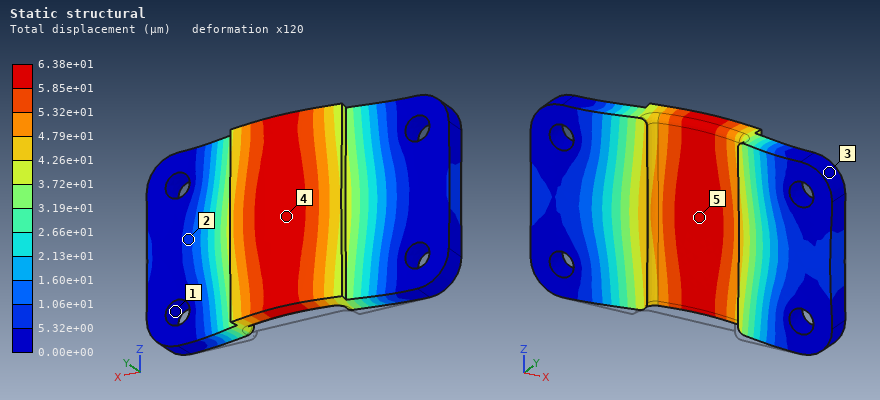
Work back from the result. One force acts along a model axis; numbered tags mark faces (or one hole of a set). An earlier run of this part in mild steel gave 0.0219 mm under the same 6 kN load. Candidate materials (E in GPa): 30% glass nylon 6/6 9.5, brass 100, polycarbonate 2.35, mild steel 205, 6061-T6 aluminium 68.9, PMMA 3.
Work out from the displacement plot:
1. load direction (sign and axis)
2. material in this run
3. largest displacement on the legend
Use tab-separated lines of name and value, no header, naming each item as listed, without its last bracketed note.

load direction	+Y
material in this run	6061-T6 aluminium
largest displacement on the legend	6.38e+01 µm
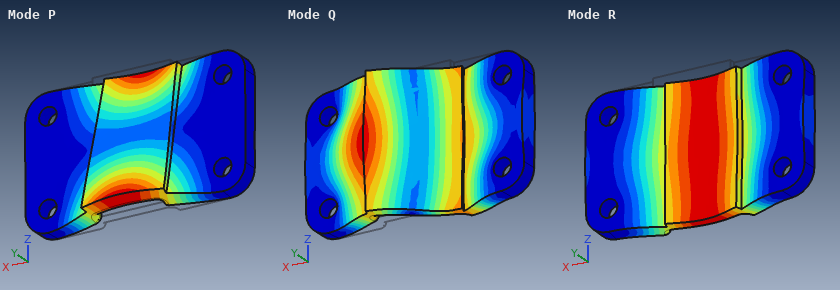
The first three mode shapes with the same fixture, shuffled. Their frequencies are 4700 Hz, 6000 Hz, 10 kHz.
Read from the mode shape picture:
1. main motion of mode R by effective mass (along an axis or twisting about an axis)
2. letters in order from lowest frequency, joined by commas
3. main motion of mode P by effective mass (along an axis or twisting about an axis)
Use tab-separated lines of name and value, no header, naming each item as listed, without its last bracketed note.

main motion of mode R by effective mass	along Y
letters in order from lowest frequency, joined by commas	R, P, Q
main motion of mode P by effective mass	twisting about X
